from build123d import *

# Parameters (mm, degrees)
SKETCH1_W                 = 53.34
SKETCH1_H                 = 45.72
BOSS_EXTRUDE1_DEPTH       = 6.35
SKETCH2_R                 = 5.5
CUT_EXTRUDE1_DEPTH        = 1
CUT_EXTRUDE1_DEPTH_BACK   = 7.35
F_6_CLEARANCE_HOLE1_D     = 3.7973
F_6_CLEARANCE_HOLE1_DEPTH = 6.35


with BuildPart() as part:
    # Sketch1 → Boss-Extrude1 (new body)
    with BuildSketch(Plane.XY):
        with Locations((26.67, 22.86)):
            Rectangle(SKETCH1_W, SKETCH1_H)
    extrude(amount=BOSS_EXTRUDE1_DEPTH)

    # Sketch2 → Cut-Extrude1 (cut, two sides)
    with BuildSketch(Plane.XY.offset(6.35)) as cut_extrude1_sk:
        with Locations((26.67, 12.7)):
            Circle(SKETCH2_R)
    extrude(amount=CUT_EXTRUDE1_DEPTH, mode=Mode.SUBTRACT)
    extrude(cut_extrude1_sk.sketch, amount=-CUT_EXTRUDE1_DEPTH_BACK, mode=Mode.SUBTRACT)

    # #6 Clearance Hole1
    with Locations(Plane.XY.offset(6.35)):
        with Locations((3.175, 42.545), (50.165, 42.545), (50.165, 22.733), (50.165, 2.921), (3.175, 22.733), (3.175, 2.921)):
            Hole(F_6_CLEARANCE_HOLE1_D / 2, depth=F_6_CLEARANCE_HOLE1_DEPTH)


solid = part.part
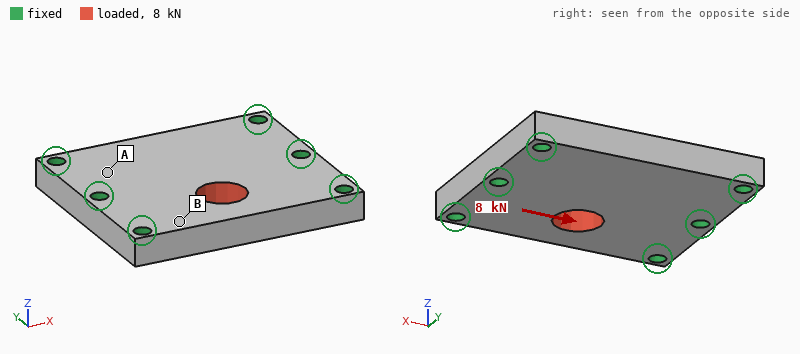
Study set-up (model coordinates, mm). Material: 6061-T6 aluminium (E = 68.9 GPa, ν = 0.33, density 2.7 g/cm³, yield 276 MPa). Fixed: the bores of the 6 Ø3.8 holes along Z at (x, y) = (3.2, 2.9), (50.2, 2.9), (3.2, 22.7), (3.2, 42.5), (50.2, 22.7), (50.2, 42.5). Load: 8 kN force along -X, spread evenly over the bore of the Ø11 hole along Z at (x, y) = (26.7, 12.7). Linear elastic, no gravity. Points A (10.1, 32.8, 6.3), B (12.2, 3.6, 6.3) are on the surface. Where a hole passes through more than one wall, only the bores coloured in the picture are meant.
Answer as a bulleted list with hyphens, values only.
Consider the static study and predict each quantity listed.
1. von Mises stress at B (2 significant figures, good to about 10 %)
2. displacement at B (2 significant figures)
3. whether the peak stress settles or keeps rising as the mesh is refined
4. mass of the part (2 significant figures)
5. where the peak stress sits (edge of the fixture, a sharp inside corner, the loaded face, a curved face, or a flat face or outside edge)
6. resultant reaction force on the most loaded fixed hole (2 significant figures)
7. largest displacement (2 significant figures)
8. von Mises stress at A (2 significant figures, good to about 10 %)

- 28 MPa
- 3.8 µm
- keeps rising
- 39 g
- edge of the fixture
- 2.0 kN
- 10 µm
- 7.3 MPa
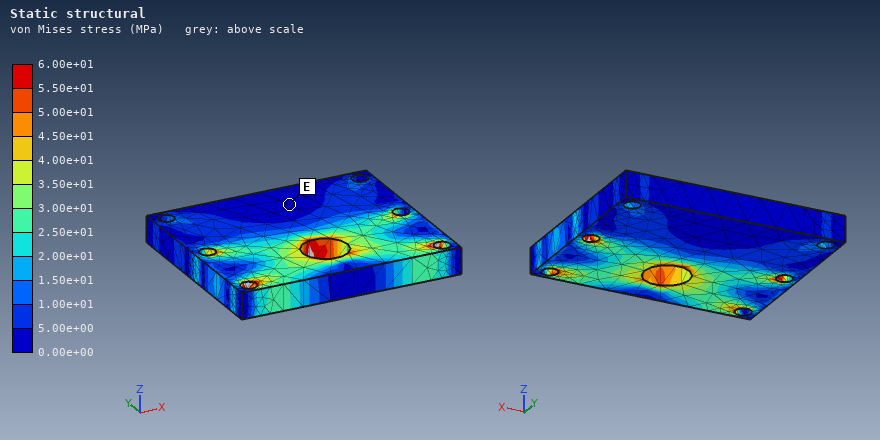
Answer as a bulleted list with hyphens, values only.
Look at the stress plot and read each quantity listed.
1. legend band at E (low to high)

- 0.00e+00 to 5.00e+00 MPa
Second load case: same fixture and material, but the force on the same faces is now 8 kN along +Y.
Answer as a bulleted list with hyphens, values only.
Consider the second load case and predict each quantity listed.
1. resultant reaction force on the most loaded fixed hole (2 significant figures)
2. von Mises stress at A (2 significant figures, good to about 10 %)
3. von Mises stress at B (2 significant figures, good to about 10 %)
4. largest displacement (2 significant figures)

- 2.0 kN
- 26 MPa
- 20 MPa
- 22 µm
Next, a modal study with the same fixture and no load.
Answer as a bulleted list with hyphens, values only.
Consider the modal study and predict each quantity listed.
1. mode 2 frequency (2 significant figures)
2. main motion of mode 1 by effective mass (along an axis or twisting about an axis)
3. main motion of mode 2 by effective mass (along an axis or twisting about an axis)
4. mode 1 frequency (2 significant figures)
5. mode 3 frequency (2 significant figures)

- 16 kHz
- along Z
- twisting about X
- 13 kHz
- 25 kHz
